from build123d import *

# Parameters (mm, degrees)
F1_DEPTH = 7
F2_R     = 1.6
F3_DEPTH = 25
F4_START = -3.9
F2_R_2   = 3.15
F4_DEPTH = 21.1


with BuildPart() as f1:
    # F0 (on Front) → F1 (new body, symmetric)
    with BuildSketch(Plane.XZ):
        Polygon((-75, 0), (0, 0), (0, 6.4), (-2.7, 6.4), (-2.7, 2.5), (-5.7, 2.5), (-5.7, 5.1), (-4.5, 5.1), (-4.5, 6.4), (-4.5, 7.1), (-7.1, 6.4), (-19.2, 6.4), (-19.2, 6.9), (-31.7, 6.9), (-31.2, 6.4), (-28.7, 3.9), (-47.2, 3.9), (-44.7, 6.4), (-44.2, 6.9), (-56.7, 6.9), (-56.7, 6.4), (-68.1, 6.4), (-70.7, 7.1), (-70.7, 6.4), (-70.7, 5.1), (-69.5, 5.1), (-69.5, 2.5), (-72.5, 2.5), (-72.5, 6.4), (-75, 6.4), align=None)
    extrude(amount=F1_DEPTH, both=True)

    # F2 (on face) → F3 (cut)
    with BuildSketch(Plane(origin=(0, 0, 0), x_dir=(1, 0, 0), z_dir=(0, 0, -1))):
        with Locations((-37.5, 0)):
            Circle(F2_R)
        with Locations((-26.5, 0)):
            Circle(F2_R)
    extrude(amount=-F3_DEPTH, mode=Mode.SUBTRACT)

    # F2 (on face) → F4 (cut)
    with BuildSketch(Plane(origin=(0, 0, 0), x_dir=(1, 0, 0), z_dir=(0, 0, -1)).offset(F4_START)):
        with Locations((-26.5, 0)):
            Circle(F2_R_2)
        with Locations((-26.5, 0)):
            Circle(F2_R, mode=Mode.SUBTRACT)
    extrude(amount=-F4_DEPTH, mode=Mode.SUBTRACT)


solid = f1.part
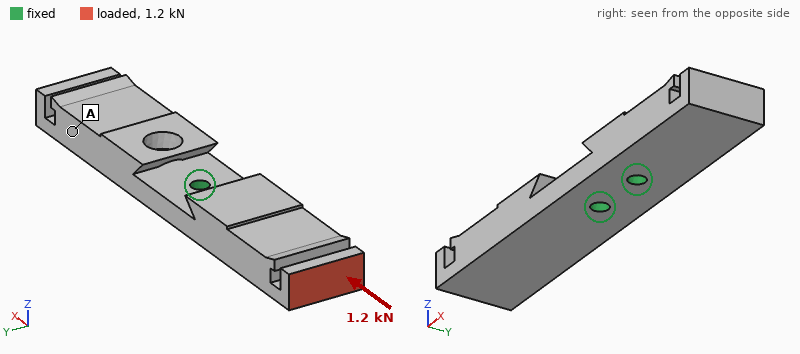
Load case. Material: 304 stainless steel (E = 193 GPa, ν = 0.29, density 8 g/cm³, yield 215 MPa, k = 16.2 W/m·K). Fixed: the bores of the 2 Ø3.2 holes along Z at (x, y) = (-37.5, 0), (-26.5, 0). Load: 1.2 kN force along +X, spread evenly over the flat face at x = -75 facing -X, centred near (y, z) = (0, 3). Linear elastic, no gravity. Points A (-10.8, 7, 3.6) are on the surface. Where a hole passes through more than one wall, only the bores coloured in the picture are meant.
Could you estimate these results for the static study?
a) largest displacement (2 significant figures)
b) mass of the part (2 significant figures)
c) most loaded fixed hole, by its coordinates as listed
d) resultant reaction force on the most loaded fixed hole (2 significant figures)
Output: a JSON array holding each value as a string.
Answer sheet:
["57 µm", "47 g", "(-37.5, 0)", "990 N"]
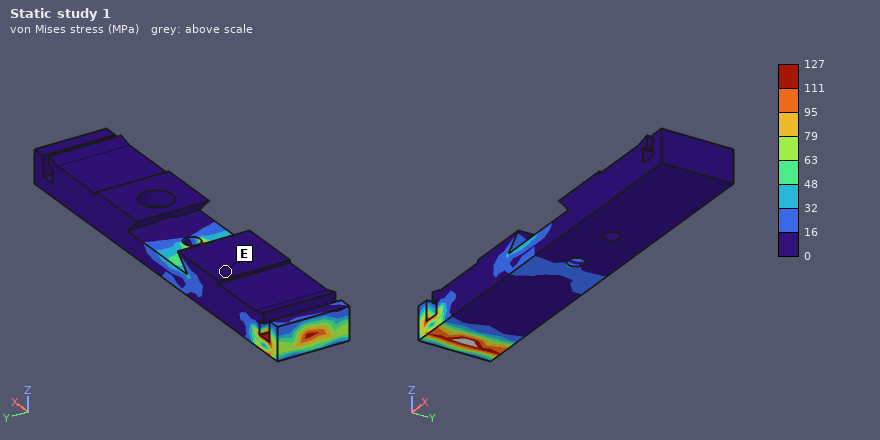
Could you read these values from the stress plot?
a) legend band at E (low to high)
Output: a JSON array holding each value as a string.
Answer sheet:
["0 to 16 MPa"]
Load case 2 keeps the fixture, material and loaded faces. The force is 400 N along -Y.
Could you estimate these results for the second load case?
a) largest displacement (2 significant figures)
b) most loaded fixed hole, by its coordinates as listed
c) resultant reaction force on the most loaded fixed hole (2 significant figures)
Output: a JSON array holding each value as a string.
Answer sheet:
["61 µm", "(-37.5, 0)", "1.3 kN"]
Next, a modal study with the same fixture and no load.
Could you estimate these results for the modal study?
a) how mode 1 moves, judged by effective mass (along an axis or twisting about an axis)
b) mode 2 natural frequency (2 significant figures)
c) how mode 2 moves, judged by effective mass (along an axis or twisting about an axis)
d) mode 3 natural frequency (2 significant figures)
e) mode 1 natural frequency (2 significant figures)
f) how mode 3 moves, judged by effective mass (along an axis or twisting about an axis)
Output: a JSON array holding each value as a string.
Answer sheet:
["along Z", "4900 Hz", "along Y", "5600 Hz", "2000 Hz", "along Z"]
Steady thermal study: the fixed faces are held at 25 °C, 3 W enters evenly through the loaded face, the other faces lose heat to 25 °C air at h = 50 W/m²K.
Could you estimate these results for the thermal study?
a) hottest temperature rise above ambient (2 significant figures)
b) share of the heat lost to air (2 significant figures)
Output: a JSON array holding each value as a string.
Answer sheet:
["64 K", "69 %"]
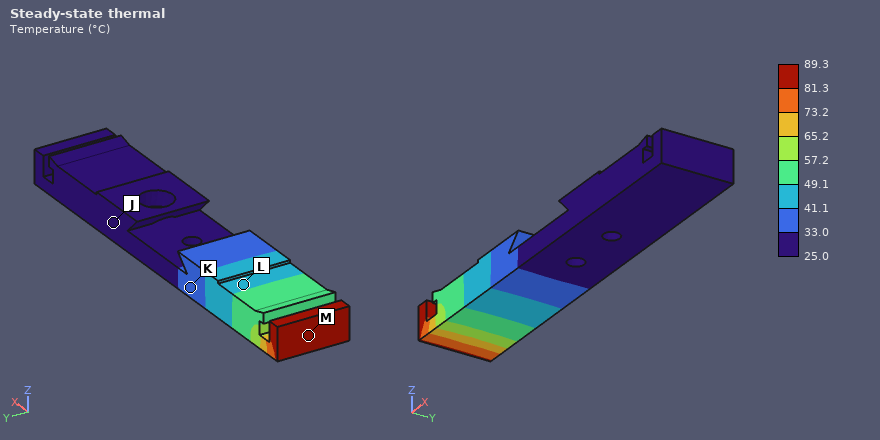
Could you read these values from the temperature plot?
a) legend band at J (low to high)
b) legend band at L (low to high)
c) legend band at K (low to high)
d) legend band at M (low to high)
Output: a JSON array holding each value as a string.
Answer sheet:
["25.0 to 33.0 °C", "41.1 to 49.1 °C", "33.0 to 41.1 °C", "81.3 to 89.3 °C"]
